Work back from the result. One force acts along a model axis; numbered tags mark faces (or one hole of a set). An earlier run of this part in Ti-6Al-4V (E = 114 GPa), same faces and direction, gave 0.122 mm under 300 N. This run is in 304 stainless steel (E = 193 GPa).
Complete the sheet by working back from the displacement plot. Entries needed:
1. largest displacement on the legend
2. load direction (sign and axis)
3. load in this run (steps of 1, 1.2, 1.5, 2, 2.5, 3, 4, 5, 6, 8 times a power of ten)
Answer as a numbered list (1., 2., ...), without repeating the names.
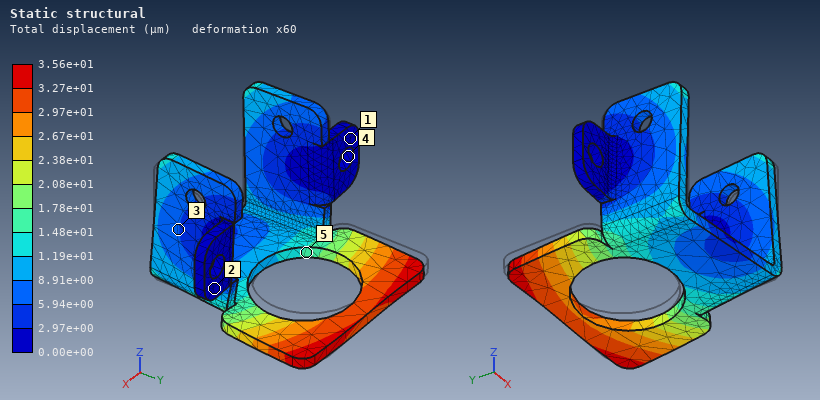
1. 3.56e+01 µm
2. +X
3. 150 N
